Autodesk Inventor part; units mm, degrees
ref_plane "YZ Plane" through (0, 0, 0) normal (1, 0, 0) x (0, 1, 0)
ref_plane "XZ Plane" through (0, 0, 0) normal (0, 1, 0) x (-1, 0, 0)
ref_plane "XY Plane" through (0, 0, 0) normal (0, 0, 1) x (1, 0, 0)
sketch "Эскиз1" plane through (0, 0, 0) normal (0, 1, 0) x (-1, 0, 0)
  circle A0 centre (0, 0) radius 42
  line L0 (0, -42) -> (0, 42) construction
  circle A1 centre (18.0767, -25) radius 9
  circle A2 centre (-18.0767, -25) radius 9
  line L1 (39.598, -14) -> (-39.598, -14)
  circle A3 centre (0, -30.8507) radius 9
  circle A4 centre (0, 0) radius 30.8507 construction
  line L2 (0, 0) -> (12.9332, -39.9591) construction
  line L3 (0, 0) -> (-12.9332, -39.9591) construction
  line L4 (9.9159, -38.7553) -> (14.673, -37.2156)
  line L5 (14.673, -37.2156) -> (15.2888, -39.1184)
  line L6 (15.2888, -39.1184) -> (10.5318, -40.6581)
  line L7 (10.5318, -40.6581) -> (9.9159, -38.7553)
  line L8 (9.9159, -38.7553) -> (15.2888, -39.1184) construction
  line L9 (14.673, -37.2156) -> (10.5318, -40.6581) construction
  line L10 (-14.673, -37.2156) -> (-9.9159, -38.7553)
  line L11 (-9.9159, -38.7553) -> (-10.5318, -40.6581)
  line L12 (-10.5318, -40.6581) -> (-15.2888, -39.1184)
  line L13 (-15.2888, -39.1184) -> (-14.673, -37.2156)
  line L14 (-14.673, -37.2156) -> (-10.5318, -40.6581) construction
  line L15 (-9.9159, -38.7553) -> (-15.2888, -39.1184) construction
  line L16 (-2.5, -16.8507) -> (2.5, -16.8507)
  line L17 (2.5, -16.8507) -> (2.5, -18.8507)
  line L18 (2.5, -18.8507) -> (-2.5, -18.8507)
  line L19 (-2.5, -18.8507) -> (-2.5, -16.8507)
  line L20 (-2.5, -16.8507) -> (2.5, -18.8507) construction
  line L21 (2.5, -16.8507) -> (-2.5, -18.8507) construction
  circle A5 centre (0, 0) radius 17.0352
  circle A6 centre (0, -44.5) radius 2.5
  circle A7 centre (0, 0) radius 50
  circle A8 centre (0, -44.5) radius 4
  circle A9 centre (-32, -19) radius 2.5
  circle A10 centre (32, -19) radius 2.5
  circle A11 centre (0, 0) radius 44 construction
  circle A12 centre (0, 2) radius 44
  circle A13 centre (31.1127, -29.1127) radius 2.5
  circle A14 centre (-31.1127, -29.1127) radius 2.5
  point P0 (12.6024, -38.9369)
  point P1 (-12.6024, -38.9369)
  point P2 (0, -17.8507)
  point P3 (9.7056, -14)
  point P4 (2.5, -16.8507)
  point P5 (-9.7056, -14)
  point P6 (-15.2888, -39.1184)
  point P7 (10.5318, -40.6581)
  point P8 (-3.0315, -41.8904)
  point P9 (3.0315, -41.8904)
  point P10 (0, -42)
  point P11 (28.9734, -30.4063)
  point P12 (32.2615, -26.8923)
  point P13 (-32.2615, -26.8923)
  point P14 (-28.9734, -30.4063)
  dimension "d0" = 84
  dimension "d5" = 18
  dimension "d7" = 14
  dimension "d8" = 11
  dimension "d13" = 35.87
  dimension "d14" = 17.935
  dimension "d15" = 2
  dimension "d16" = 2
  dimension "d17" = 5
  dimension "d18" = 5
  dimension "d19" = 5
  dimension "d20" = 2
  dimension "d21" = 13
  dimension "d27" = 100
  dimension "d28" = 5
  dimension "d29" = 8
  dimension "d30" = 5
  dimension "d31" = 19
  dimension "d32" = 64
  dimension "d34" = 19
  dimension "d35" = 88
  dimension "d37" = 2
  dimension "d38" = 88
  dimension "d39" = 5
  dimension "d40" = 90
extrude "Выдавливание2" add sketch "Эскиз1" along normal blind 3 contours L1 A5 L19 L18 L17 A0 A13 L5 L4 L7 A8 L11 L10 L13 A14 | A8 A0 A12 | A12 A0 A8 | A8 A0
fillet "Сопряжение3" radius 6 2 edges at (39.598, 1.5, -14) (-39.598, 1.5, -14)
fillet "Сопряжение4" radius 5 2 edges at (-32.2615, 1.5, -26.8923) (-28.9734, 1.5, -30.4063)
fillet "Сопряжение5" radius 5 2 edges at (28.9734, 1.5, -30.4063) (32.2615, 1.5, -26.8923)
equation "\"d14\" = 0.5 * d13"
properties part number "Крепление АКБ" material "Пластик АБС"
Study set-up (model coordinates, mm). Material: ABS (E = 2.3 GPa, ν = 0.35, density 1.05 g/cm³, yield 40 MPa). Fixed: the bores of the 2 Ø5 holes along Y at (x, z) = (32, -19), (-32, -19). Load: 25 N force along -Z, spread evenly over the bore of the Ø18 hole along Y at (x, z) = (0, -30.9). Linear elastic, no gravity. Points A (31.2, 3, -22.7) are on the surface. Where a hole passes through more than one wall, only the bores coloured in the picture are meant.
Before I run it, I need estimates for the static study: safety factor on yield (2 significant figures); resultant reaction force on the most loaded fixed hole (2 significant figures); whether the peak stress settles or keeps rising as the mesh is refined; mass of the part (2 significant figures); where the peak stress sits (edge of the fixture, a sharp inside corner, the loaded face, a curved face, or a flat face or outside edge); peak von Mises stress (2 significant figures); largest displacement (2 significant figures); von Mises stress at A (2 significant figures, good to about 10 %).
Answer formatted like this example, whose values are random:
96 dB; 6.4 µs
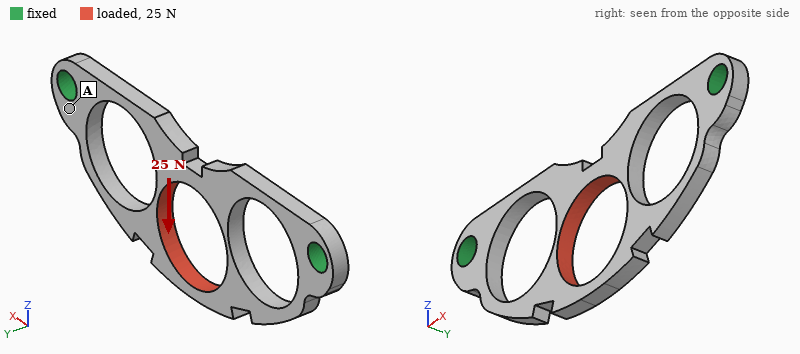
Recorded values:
4.9; 19 N; settles; 2.1 g; a curved face; 8.2 MPa; 0.14 mm; 1.3 MPa
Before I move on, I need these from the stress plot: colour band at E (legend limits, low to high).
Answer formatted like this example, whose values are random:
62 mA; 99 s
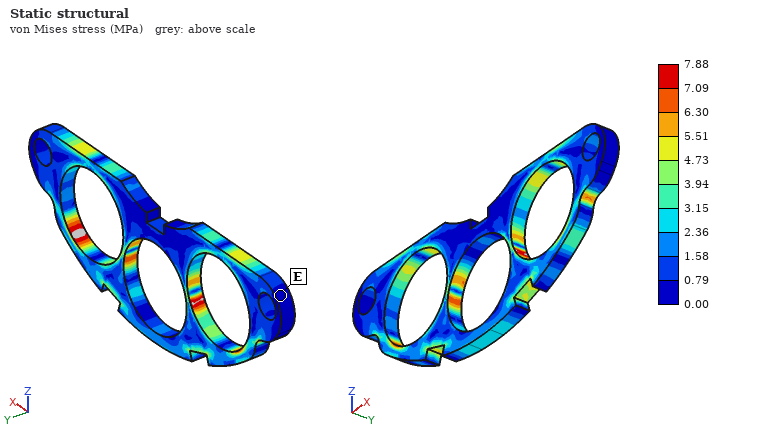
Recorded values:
0.00 to 0.79 MPa
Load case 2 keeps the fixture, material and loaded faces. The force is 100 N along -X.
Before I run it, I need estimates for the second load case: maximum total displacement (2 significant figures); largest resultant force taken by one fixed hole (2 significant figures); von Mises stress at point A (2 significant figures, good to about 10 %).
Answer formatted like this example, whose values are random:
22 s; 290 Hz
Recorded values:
0.20 mm; 54 N; 3.3 MPa
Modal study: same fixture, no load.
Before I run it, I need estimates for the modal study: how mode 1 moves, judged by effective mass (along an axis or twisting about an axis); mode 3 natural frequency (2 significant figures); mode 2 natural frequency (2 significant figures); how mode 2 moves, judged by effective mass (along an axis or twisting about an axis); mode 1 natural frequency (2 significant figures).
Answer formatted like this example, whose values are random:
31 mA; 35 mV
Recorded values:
along Y; 1900 Hz; 1300 Hz; along Y; 640 Hz
